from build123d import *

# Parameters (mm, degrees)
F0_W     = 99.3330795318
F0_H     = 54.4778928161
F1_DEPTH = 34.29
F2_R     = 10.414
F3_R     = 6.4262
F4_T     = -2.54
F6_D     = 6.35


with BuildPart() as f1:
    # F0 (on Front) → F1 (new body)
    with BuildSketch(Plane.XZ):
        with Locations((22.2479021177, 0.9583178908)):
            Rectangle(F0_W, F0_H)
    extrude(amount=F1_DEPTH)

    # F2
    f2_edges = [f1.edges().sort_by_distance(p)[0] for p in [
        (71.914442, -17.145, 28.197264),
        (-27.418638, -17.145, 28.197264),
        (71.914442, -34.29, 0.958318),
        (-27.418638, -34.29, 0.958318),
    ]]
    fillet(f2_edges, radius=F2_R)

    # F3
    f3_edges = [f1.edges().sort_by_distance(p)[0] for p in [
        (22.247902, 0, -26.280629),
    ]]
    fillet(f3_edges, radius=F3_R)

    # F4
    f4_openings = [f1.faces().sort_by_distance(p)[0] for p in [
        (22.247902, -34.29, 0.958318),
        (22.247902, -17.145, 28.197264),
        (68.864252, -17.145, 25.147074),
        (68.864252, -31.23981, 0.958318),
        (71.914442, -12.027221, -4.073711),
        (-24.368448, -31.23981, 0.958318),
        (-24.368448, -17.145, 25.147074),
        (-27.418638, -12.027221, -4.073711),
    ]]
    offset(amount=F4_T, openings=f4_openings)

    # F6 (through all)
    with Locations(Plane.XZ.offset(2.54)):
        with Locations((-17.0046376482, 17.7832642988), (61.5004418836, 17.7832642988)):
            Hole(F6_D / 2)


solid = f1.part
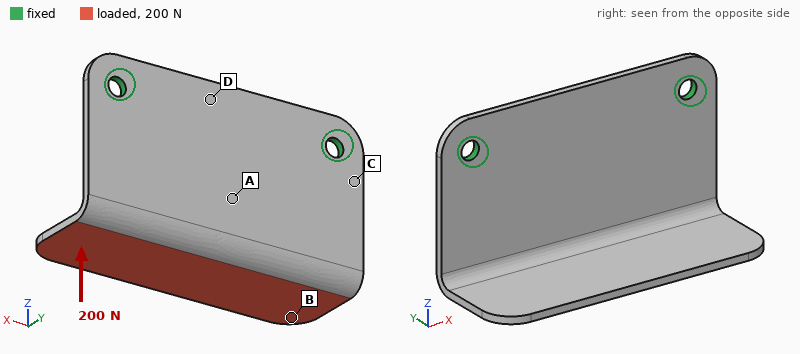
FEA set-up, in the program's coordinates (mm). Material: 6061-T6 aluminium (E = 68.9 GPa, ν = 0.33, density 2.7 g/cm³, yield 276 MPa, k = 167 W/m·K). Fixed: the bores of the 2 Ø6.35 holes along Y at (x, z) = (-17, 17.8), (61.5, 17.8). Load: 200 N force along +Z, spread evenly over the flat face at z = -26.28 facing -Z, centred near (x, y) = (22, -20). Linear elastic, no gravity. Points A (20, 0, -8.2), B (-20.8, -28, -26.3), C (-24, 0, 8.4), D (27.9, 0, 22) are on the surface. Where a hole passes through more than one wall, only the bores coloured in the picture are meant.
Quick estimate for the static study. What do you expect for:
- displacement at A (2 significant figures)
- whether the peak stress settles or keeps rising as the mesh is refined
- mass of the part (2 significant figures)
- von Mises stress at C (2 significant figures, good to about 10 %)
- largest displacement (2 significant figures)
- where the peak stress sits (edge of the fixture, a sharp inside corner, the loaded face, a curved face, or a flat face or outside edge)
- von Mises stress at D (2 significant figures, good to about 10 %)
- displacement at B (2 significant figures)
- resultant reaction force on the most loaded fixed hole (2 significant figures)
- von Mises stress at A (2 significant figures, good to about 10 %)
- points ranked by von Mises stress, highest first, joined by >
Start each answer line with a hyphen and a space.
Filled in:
- 0.18 mm
- keeps rising
- 56 g
- 49 MPa
- 0.81 mm
- edge of the fixture
- 11 MPa
- 0.70 mm
- 110 N
- 28 MPa
- C > A > D > B
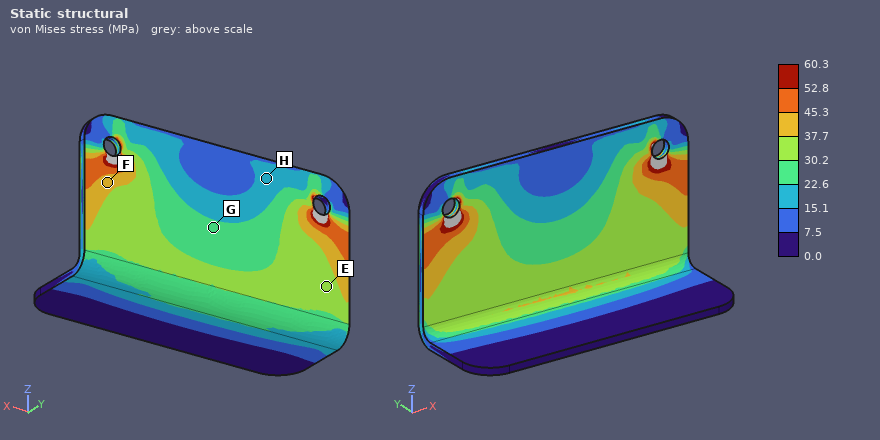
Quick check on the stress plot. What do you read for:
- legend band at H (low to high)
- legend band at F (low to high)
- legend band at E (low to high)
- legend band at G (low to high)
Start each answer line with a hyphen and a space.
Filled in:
- 15.1 to 22.6 MPa
- 37.7 to 45.3 MPa
- 30.2 to 37.7 MPa
- 22.6 to 30.2 MPa
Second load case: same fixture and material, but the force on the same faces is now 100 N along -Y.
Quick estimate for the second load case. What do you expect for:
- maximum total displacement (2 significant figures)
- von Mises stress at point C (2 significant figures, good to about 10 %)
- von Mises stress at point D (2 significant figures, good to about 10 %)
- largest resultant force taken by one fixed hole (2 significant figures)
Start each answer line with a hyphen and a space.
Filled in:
- 0.55 mm
- 50 MPa
- 7.1 MPa
- 51 N
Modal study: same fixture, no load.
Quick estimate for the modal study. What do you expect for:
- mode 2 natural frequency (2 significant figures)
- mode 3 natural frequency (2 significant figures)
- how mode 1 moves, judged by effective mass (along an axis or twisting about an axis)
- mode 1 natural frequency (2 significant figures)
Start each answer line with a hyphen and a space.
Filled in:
- 860 Hz
- 1400 Hz
- along Y
- 440 Hz
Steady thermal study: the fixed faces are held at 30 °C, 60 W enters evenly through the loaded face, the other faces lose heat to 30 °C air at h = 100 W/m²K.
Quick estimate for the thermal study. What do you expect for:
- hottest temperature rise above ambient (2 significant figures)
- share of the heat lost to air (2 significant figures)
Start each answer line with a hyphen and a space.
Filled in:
- 55 K
- 62 %
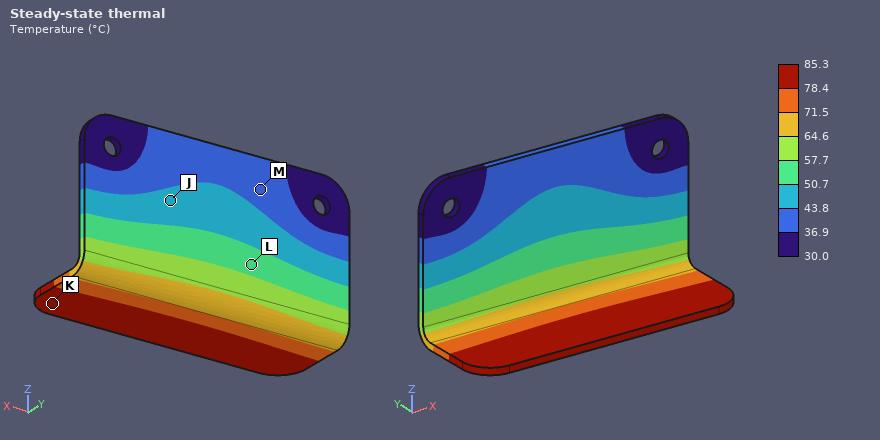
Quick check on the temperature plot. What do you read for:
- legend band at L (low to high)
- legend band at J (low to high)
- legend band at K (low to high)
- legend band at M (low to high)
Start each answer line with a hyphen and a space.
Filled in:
- 50.7 to 57.7 °C
- 43.8 to 50.7 °C
- 78.4 to 85.3 °C
- 36.9 to 43.8 °C
